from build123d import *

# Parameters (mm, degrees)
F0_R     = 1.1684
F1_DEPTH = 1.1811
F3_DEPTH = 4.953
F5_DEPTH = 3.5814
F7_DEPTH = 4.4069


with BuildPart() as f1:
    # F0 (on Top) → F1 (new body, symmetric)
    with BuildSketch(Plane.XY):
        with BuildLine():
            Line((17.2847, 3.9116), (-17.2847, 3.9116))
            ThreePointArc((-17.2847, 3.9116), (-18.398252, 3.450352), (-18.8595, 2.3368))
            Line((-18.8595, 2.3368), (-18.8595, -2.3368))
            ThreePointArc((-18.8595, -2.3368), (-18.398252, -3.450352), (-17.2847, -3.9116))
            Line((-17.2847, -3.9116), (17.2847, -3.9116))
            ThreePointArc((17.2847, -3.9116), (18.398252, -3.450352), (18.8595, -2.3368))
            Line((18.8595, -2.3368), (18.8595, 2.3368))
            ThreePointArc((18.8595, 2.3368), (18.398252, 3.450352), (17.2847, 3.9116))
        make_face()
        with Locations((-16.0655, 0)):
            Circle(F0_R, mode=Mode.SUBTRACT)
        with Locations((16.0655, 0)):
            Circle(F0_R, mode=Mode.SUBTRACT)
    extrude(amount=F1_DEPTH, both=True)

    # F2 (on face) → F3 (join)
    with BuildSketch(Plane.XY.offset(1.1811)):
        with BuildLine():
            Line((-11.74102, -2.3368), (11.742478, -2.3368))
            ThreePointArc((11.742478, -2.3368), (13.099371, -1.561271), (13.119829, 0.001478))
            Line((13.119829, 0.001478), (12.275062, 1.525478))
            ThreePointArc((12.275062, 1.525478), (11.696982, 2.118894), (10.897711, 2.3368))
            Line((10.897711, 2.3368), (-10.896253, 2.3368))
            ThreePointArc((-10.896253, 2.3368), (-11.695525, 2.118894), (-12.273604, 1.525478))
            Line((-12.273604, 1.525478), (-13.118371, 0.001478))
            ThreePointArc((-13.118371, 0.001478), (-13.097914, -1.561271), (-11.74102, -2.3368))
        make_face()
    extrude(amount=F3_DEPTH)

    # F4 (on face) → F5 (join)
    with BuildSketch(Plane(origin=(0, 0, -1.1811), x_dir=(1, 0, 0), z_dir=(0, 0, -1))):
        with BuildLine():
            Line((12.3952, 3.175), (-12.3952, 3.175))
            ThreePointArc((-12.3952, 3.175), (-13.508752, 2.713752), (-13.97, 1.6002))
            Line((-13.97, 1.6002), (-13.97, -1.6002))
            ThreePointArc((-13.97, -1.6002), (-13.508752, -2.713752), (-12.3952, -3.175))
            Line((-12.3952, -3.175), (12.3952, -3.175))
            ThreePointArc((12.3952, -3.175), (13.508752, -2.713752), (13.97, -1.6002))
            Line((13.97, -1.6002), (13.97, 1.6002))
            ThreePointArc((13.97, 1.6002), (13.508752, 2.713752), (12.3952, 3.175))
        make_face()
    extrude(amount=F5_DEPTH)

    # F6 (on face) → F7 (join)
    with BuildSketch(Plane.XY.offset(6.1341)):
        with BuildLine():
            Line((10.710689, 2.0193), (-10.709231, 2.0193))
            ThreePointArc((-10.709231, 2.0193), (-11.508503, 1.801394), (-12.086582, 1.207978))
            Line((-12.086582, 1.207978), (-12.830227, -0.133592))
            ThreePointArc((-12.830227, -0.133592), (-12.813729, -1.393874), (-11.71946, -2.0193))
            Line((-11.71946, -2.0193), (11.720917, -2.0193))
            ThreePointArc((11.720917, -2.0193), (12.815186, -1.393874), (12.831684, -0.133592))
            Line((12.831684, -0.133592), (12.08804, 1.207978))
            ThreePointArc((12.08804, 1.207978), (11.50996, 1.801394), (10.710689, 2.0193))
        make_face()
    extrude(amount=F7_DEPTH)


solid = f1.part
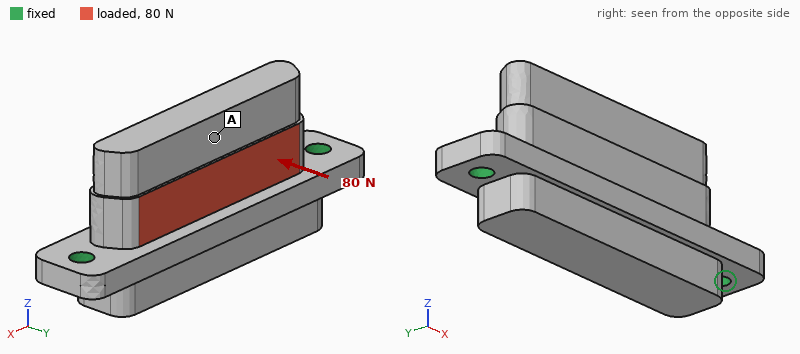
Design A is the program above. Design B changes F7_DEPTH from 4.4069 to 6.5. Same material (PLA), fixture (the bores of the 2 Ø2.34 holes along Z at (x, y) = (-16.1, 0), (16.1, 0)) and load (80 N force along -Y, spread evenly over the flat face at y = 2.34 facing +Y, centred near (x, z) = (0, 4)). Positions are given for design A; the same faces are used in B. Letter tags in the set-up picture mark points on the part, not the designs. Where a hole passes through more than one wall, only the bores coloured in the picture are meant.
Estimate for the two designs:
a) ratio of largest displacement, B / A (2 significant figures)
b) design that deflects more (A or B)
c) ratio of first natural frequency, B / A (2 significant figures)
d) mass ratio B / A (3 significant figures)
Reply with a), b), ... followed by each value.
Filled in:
a) 1.1
b) B
c) 0.80
d) 1.09
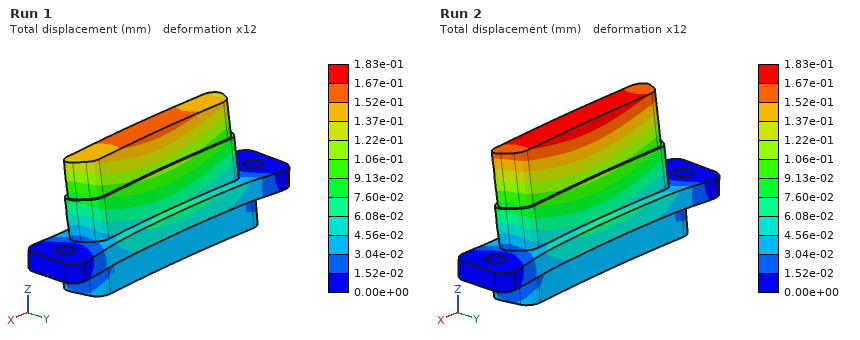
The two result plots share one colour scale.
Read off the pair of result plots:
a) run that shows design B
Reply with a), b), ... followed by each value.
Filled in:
a) Run 2
